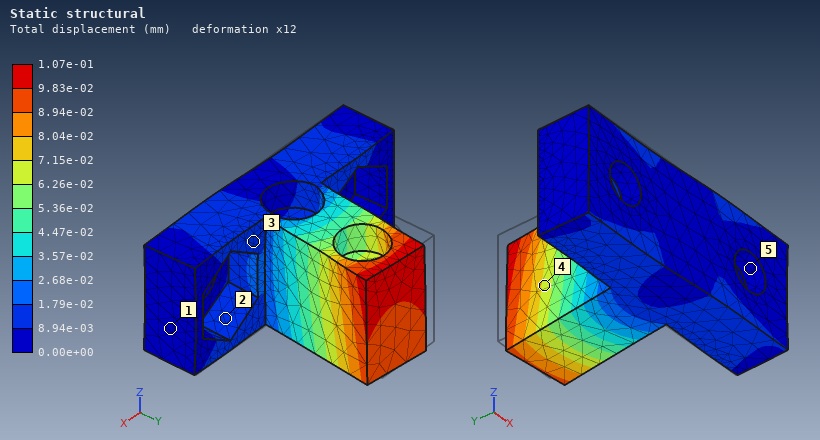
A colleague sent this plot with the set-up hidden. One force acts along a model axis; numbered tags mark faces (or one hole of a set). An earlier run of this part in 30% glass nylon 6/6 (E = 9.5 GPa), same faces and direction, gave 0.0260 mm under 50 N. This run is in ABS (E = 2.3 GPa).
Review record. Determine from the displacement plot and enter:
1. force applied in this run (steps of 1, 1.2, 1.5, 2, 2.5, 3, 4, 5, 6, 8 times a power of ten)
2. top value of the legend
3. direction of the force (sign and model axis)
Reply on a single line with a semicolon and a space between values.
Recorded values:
50 N; 1.07e-01 mm; +X
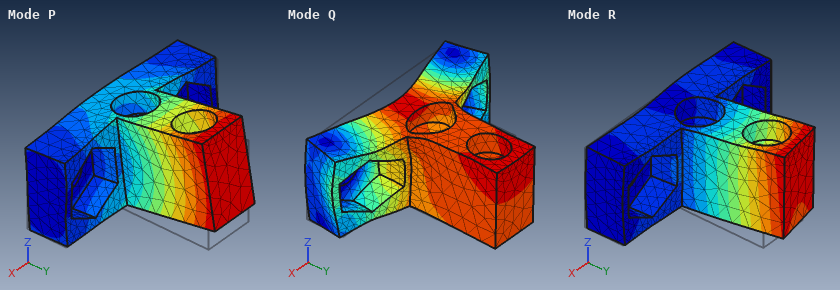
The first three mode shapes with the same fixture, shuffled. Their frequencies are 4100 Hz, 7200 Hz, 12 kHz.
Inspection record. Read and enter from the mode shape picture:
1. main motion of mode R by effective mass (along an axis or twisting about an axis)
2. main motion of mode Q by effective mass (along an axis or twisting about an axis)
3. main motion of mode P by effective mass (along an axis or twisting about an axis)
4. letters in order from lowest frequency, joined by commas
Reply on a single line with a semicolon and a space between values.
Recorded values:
along X; along Y; along Z; P, R, Q
